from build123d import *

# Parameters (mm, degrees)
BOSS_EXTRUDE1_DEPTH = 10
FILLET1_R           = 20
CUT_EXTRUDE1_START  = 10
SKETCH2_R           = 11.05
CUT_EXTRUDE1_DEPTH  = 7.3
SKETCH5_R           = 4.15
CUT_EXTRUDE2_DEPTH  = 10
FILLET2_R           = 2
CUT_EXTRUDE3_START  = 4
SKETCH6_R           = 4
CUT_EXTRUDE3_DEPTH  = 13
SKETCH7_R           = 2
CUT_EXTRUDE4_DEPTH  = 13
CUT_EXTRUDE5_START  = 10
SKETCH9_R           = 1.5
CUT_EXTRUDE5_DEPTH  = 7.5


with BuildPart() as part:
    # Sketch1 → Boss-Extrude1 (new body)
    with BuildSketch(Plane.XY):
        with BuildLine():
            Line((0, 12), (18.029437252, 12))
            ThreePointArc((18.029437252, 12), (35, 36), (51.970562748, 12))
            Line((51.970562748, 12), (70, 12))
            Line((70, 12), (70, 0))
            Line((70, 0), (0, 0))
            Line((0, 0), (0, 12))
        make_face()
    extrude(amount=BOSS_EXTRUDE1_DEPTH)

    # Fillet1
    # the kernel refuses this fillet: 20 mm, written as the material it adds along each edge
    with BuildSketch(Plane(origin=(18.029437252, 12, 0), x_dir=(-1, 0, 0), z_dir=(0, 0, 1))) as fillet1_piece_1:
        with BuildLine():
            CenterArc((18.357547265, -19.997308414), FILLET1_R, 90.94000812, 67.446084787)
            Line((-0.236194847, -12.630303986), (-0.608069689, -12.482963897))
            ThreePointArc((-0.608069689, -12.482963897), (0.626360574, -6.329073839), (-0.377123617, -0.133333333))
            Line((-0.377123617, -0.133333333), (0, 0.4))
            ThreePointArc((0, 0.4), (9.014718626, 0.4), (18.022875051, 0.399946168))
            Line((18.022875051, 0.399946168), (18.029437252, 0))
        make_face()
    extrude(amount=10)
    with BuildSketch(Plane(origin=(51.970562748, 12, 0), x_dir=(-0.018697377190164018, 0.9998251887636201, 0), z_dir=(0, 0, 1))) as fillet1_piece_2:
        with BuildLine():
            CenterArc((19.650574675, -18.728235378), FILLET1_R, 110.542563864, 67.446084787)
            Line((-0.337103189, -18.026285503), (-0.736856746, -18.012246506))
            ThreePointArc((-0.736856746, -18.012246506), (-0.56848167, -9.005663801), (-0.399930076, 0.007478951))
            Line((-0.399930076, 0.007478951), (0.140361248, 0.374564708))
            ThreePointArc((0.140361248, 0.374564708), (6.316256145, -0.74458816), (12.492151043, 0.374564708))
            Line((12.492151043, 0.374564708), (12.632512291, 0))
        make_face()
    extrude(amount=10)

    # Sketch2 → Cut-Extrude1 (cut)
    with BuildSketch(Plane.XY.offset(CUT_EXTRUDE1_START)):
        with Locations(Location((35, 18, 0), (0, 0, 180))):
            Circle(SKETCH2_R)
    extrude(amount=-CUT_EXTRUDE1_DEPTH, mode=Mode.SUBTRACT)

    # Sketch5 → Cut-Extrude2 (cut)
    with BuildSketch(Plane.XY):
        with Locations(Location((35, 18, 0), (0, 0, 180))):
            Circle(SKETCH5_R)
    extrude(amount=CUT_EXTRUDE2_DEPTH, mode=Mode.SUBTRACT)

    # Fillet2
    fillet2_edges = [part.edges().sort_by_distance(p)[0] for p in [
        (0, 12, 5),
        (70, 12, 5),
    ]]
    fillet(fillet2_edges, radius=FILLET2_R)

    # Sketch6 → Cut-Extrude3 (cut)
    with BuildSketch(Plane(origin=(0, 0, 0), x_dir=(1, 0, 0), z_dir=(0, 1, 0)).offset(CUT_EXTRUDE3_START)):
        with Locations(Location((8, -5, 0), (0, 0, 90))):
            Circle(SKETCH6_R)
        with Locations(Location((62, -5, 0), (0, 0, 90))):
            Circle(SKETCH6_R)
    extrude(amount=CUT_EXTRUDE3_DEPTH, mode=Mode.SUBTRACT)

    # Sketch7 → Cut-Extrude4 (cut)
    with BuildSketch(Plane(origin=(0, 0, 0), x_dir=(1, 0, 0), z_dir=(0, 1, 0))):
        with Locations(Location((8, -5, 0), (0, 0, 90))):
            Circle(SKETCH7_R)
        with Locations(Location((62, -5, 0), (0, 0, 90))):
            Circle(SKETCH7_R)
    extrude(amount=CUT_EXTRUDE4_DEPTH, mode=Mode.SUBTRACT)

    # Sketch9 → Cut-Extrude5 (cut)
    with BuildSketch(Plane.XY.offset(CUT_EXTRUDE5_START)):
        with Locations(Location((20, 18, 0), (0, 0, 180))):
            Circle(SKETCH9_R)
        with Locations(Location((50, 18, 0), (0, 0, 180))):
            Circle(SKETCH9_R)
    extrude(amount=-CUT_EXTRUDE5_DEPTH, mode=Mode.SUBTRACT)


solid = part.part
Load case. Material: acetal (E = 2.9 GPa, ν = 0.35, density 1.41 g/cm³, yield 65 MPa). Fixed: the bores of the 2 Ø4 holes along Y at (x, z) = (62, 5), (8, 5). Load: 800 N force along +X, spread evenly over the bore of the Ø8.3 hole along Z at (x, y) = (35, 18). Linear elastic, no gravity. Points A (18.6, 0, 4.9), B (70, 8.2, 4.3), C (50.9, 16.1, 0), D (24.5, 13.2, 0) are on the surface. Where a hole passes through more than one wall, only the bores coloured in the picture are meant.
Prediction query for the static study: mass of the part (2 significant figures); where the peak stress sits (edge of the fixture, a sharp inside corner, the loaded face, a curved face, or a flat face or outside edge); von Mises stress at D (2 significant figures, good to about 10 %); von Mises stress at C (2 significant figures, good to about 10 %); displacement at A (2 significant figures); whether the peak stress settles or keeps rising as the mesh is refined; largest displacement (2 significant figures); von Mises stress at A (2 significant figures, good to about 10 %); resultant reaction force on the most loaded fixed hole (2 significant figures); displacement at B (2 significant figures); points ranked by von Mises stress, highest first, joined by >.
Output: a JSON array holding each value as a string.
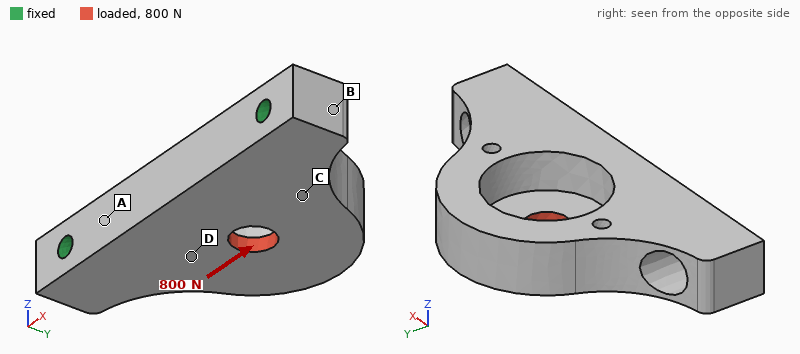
["18 g", "edge of the fixture", "9.2 MPa", "6.5 MPa", "0.020 mm", "keeps rising", "0.13 mm", "3.9 MPa", "470 N", "0.036 mm", "D > C > A > B"]
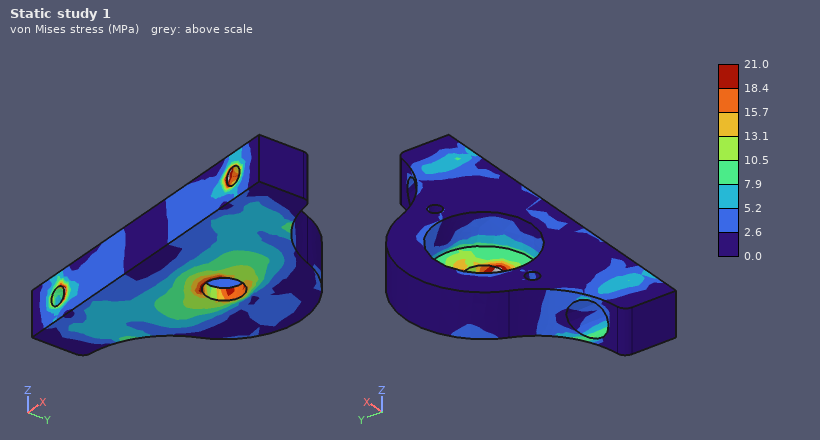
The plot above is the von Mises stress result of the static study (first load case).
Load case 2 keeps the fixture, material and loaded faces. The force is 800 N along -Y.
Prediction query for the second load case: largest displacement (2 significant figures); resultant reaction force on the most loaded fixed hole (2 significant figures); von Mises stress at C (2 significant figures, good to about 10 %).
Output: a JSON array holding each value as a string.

["0.66 mm", "480 N", "7.5 MPa"]
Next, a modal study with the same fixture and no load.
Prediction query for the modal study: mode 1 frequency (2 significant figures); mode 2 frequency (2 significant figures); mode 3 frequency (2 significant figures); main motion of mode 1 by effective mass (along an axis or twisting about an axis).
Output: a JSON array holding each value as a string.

["1000 Hz", "3400 Hz", "3500 Hz", "along Z"]
